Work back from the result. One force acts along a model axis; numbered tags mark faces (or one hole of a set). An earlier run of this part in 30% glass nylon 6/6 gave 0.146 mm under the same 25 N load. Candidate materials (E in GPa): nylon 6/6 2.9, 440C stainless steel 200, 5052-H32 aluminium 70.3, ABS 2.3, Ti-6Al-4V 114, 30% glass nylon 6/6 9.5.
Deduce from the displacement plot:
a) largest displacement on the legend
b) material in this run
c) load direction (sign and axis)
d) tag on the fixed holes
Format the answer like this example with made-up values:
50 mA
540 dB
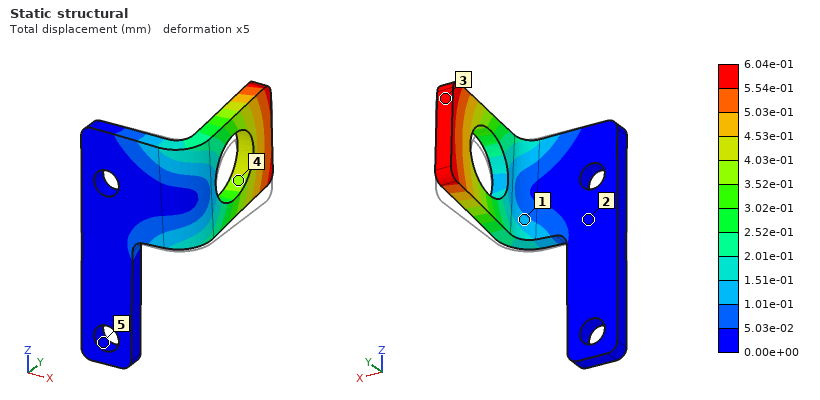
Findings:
6.04e-01 mm
ABS
+Z
5
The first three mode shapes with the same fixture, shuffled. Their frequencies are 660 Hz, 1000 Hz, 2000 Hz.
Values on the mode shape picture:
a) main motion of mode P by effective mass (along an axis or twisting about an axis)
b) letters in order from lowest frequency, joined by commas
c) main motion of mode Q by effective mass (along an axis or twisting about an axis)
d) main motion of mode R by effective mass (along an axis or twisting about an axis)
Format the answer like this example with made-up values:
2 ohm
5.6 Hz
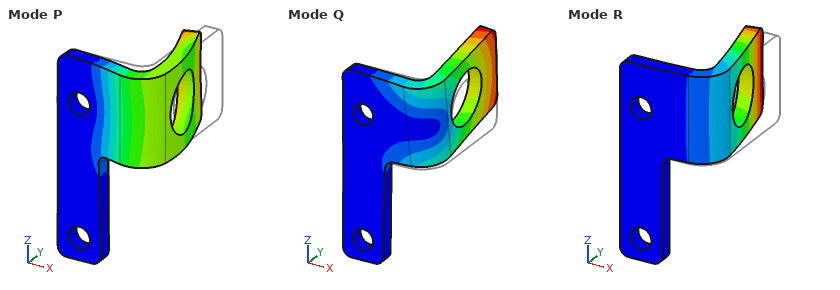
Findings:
along Y
R, Q, P
along Z
along X
